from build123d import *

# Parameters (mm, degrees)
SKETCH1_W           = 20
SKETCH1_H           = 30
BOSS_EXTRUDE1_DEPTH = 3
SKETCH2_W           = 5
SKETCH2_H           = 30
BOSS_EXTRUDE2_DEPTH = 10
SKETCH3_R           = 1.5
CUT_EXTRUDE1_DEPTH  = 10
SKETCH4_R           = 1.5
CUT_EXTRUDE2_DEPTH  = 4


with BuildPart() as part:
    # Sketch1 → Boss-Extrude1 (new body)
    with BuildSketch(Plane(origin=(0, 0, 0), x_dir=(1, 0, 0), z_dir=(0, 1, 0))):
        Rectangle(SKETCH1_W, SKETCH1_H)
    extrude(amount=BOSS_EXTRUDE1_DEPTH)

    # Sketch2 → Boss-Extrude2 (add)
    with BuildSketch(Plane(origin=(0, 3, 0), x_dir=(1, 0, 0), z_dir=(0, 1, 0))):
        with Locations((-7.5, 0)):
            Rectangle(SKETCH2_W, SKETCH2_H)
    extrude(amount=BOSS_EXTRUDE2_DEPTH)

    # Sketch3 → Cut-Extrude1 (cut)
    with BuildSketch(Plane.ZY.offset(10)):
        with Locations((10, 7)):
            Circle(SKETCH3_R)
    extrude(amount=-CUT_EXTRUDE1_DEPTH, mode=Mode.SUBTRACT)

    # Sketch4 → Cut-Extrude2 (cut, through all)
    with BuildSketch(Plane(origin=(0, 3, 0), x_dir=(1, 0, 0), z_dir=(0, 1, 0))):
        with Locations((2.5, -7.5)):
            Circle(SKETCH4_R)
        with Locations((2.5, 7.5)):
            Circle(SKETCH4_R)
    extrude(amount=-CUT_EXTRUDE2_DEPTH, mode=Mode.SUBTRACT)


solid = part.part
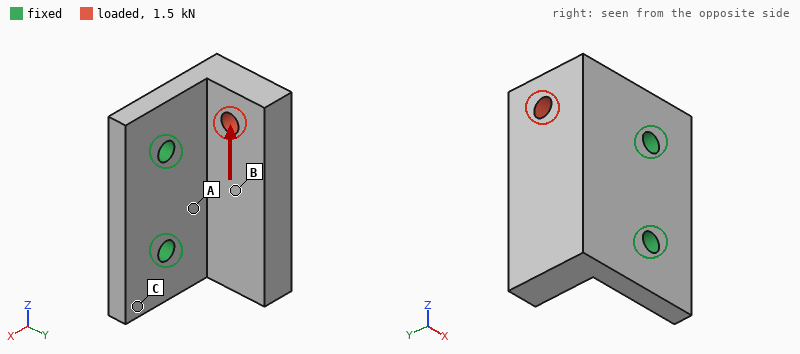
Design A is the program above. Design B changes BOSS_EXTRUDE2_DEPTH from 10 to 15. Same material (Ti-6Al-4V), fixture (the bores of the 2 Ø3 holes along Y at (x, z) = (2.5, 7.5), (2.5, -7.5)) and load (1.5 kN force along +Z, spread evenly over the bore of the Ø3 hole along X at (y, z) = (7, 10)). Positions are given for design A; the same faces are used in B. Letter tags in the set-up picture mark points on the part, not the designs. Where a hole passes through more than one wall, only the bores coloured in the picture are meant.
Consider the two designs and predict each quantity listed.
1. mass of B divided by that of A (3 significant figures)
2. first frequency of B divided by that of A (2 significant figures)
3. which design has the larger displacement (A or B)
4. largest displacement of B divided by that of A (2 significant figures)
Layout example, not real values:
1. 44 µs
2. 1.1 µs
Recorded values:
1. 1.23
2. 0.68
3. B
4. 1.1
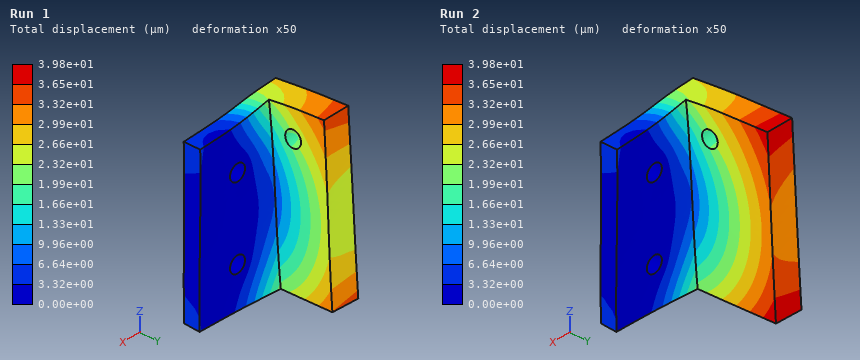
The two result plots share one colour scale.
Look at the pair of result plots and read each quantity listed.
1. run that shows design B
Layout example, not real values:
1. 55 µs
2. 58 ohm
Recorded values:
1. Run 2
